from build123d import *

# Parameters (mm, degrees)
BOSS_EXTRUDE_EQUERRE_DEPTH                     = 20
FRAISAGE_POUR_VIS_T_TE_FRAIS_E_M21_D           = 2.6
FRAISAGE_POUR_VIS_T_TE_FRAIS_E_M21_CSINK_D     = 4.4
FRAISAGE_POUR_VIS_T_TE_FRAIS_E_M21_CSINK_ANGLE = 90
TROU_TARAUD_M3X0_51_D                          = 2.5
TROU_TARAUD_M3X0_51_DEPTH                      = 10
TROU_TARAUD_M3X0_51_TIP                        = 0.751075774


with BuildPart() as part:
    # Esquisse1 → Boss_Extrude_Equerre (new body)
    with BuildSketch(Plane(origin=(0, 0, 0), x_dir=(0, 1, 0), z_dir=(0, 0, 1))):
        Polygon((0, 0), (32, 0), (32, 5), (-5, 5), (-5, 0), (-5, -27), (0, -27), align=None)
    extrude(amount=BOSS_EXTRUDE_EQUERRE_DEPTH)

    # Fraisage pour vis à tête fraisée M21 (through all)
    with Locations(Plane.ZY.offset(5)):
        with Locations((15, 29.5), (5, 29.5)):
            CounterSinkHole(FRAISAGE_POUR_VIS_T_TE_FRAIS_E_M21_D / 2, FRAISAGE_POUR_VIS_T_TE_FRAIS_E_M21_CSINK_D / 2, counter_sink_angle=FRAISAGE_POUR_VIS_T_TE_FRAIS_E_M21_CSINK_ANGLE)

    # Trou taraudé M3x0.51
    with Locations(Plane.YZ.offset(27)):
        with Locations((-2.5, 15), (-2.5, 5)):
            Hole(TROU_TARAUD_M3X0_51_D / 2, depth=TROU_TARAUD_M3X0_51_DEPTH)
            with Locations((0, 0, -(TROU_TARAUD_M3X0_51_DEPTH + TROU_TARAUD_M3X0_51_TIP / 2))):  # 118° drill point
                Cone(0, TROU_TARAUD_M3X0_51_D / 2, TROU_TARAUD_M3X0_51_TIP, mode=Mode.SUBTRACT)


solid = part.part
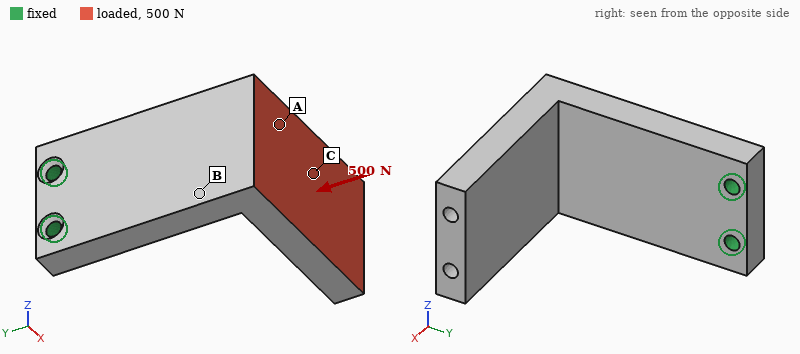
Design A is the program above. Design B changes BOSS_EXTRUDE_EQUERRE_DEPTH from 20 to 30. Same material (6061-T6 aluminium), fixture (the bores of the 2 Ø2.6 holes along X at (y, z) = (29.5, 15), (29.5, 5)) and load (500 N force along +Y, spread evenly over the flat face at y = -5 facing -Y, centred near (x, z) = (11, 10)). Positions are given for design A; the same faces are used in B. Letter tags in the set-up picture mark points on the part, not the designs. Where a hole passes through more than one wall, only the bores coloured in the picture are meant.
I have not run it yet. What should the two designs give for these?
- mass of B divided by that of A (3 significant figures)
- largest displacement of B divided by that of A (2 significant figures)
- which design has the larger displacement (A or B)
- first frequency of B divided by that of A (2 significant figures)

1.51
0.73
A
0.91
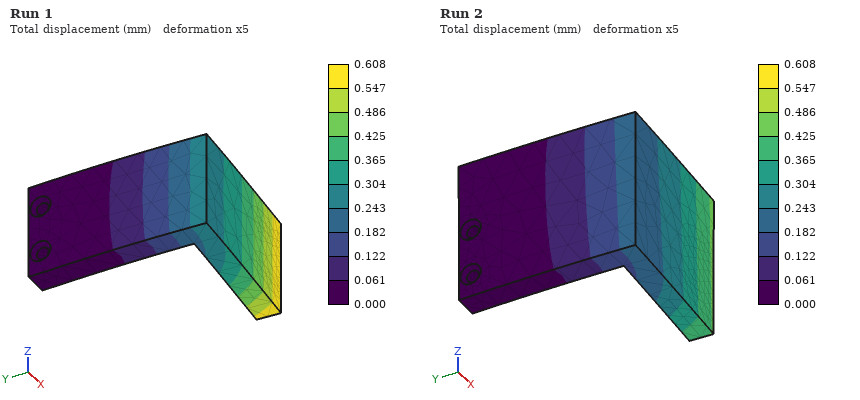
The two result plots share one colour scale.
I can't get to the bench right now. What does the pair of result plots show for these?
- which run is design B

Run 2
